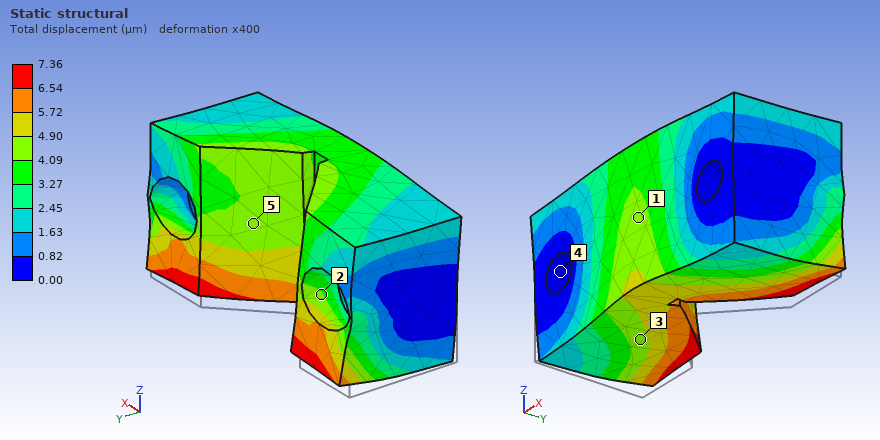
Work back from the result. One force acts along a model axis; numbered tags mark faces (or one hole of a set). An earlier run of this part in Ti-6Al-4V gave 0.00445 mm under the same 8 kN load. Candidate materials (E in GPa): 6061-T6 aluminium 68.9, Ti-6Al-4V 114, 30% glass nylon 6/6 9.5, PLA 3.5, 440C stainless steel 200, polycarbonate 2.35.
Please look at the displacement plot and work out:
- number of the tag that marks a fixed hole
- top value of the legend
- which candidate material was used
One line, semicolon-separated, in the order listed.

4; 7.36 µm; 6061-T6 aluminium
